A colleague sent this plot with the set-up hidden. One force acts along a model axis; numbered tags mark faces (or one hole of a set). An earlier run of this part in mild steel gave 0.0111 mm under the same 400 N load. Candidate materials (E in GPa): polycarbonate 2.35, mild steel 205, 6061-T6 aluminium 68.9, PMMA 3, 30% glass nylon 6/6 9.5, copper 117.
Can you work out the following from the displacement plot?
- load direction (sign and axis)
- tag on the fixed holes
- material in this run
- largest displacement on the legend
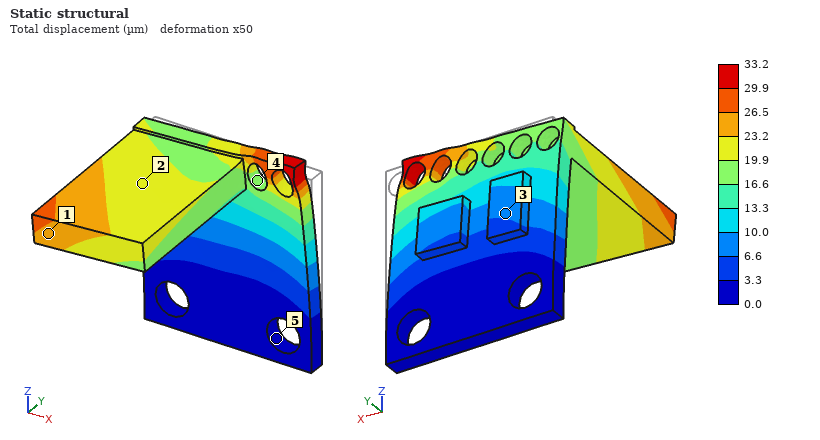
-X
5
6061-T6 aluminium
33.2 µm
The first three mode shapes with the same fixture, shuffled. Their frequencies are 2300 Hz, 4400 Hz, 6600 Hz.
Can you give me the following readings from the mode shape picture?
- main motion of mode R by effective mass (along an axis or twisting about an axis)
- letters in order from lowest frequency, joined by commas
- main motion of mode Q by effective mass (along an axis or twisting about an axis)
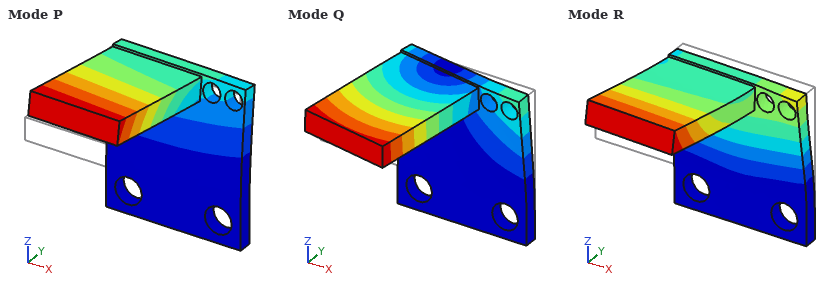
along Y
P, Q, R
along X
